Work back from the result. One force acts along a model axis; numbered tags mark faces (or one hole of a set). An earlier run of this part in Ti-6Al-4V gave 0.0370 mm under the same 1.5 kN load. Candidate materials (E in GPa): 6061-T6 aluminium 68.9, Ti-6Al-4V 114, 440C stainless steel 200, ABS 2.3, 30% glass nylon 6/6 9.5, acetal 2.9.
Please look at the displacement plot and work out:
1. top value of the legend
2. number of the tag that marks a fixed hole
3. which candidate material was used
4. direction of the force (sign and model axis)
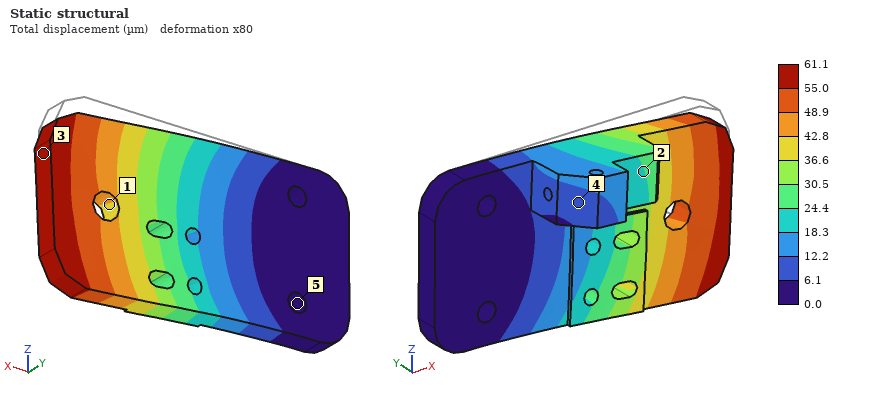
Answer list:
61.1 µm
5
6061-T6 aluminium
-Z
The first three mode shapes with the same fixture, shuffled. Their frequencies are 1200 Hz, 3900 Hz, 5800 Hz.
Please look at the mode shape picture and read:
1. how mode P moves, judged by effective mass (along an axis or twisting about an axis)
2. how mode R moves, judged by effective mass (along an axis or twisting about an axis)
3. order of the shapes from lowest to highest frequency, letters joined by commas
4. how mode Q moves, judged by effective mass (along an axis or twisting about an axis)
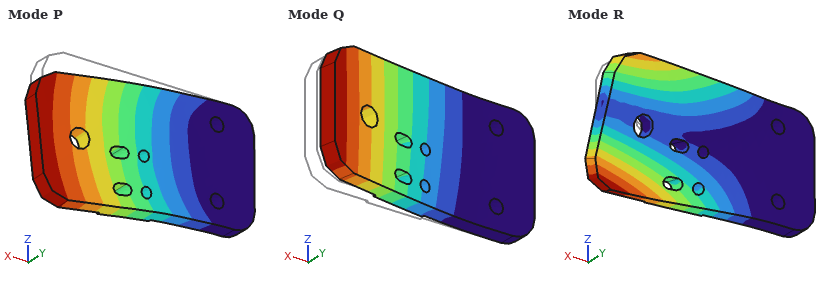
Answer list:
along Z
twisting about X
Q, R, P
along Y
